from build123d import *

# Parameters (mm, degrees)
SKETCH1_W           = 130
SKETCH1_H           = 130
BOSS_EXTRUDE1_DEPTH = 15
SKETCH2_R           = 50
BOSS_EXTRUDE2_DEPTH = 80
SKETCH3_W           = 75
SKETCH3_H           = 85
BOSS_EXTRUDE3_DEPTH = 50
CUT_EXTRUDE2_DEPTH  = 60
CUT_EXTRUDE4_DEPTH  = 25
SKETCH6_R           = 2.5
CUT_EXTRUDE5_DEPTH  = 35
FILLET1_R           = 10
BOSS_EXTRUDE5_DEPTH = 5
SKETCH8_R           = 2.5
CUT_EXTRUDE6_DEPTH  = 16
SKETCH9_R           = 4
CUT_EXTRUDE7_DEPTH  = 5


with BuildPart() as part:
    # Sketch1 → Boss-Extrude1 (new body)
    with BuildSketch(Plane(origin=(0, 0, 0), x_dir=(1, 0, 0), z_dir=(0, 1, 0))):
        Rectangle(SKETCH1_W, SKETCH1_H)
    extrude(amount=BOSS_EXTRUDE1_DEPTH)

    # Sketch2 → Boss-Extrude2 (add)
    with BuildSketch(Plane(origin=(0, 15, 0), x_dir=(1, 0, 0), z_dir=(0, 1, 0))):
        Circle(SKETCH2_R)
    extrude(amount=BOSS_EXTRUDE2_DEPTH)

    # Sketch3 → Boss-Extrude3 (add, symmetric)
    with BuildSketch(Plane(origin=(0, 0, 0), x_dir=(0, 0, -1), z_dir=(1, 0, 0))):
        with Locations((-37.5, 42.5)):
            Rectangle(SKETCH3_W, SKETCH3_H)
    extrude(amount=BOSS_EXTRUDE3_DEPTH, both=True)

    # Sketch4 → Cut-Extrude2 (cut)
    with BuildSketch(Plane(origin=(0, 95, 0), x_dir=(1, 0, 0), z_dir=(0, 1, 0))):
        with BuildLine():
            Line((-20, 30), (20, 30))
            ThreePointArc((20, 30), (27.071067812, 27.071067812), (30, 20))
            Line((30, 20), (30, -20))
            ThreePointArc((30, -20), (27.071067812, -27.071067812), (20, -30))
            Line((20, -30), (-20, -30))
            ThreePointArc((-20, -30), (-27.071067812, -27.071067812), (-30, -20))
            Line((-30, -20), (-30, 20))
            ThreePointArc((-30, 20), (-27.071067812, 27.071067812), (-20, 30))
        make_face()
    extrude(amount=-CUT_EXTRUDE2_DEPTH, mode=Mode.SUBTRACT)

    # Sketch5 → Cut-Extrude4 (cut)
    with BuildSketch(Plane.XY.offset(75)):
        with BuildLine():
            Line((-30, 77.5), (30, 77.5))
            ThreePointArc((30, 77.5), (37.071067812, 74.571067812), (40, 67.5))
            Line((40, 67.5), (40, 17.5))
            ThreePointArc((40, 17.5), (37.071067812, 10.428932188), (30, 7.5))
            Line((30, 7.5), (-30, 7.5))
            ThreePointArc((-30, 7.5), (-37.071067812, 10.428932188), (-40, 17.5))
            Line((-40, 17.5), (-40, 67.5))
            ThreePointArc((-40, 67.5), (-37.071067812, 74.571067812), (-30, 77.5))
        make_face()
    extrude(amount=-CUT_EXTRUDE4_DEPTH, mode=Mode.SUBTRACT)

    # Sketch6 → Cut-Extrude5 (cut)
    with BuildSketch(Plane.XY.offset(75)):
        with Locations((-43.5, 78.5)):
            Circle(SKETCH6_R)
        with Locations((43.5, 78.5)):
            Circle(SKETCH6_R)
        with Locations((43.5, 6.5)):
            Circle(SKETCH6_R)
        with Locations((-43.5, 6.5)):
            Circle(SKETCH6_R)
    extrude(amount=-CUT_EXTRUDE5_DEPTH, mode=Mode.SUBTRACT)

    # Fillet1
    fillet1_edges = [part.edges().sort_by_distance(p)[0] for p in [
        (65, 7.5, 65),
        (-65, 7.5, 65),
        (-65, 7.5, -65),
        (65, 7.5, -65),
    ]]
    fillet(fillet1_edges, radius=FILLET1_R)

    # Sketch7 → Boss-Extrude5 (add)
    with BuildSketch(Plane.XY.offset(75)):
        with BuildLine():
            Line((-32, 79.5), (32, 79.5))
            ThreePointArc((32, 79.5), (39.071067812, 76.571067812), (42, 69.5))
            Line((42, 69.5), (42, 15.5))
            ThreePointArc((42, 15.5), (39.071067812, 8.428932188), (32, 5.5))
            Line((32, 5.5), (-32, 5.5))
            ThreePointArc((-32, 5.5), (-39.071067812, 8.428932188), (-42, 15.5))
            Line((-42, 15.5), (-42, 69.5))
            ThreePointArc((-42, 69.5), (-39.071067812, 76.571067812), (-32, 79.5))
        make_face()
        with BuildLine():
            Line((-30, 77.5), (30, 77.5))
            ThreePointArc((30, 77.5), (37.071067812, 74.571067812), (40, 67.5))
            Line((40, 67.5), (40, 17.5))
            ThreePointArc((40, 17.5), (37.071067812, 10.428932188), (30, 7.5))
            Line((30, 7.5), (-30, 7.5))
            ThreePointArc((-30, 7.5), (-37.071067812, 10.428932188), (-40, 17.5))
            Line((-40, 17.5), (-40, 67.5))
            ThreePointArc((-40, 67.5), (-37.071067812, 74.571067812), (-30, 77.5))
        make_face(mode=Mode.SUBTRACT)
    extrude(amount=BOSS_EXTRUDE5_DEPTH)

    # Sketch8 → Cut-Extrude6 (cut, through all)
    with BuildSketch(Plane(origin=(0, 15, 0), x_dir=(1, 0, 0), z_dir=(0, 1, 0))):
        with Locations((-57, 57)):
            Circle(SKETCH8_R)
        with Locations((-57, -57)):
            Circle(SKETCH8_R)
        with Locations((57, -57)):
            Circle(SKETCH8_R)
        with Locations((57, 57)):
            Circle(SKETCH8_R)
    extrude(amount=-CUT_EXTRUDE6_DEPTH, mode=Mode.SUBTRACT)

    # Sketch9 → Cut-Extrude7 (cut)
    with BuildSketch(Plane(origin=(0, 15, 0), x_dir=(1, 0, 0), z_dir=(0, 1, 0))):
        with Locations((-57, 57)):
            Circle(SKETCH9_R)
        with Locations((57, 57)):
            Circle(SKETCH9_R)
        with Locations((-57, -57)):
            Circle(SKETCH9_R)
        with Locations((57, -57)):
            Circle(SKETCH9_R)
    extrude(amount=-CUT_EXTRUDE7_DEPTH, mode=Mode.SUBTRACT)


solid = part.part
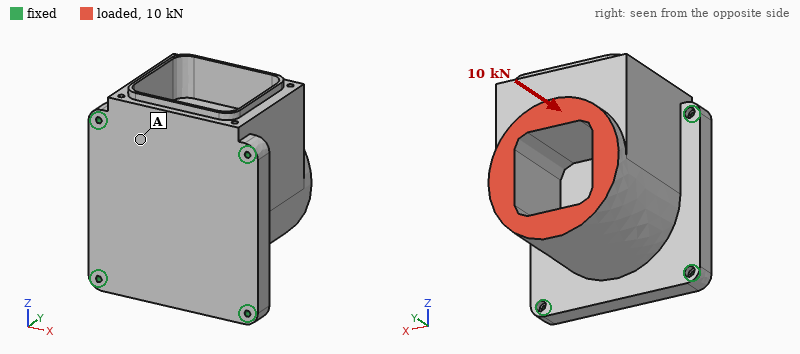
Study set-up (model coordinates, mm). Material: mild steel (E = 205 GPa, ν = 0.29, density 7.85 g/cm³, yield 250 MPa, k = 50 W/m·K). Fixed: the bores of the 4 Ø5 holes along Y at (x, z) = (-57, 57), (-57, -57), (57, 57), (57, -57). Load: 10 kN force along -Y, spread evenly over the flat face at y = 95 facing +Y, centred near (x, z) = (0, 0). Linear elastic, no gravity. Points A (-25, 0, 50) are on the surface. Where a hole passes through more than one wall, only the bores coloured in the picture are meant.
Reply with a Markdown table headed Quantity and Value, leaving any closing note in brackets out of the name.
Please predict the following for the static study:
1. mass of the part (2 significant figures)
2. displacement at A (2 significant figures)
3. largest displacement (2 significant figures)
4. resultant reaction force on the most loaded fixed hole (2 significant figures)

| Quantity | Value |
|---|---|
| mass of the part | 6.2 kg |
| displacement at A | 3.5 µm |
| largest displacement | 14 µm |
| resultant reaction force on the most loaded fixed hole | 3.1 kN |
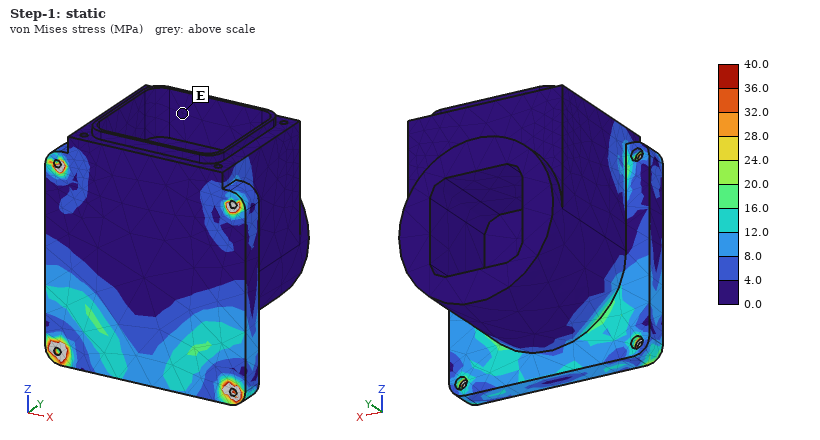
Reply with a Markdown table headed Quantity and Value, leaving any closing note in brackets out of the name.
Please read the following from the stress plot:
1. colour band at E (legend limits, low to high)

| Quantity | Value |
|---|---|
| colour band at E | 0.0 to 4.0 MPa |
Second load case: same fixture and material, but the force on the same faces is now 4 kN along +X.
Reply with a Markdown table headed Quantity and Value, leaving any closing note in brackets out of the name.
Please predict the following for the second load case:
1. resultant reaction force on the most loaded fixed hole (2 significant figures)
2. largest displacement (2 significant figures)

| Quantity | Value |
|---|---|
| resultant reaction force on the most loaded fixed hole | 2.9 kN |
| largest displacement | 9.7 µm |
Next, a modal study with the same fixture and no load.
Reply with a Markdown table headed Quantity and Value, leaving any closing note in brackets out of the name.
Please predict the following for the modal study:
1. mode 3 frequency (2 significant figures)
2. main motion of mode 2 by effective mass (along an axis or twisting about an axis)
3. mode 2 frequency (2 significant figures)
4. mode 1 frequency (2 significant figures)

| Quantity | Value |
|---|---|
| mode 3 frequency | 3400 Hz |
| main motion of mode 2 by effective mass | along X |
| mode 2 frequency | 2800 Hz |
| mode 1 frequency | 2100 Hz |
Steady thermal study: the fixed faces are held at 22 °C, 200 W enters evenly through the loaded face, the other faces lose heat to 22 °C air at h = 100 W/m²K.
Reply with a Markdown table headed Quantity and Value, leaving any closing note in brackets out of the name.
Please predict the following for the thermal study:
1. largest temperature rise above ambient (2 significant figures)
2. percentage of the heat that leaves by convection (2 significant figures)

| Quantity | Value |
|---|---|
| largest temperature rise above ambient | 54 K |
| percentage of the heat that leaves by convection | 84 % |
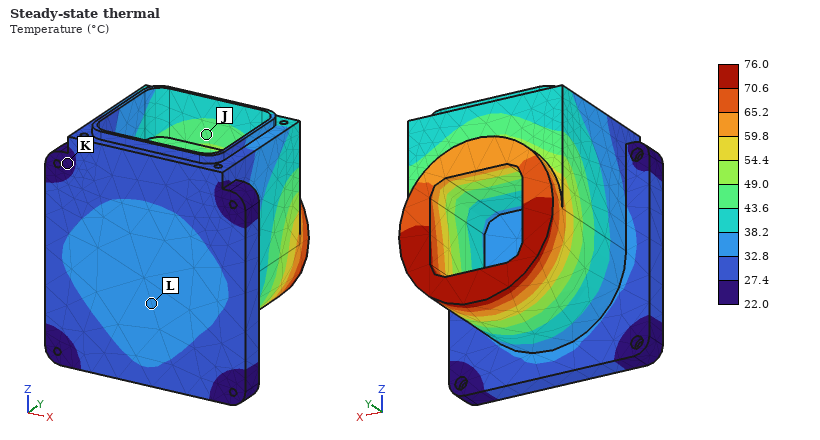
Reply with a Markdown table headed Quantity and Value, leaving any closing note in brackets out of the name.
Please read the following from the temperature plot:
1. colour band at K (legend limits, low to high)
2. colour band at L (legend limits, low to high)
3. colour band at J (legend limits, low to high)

| Quantity | Value |
|---|---|
| colour band at K | 22.0 to 27.4 °C |
| colour band at L | 32.8 to 38.2 °C |
| colour band at J | 43.6 to 49.0 °C |
